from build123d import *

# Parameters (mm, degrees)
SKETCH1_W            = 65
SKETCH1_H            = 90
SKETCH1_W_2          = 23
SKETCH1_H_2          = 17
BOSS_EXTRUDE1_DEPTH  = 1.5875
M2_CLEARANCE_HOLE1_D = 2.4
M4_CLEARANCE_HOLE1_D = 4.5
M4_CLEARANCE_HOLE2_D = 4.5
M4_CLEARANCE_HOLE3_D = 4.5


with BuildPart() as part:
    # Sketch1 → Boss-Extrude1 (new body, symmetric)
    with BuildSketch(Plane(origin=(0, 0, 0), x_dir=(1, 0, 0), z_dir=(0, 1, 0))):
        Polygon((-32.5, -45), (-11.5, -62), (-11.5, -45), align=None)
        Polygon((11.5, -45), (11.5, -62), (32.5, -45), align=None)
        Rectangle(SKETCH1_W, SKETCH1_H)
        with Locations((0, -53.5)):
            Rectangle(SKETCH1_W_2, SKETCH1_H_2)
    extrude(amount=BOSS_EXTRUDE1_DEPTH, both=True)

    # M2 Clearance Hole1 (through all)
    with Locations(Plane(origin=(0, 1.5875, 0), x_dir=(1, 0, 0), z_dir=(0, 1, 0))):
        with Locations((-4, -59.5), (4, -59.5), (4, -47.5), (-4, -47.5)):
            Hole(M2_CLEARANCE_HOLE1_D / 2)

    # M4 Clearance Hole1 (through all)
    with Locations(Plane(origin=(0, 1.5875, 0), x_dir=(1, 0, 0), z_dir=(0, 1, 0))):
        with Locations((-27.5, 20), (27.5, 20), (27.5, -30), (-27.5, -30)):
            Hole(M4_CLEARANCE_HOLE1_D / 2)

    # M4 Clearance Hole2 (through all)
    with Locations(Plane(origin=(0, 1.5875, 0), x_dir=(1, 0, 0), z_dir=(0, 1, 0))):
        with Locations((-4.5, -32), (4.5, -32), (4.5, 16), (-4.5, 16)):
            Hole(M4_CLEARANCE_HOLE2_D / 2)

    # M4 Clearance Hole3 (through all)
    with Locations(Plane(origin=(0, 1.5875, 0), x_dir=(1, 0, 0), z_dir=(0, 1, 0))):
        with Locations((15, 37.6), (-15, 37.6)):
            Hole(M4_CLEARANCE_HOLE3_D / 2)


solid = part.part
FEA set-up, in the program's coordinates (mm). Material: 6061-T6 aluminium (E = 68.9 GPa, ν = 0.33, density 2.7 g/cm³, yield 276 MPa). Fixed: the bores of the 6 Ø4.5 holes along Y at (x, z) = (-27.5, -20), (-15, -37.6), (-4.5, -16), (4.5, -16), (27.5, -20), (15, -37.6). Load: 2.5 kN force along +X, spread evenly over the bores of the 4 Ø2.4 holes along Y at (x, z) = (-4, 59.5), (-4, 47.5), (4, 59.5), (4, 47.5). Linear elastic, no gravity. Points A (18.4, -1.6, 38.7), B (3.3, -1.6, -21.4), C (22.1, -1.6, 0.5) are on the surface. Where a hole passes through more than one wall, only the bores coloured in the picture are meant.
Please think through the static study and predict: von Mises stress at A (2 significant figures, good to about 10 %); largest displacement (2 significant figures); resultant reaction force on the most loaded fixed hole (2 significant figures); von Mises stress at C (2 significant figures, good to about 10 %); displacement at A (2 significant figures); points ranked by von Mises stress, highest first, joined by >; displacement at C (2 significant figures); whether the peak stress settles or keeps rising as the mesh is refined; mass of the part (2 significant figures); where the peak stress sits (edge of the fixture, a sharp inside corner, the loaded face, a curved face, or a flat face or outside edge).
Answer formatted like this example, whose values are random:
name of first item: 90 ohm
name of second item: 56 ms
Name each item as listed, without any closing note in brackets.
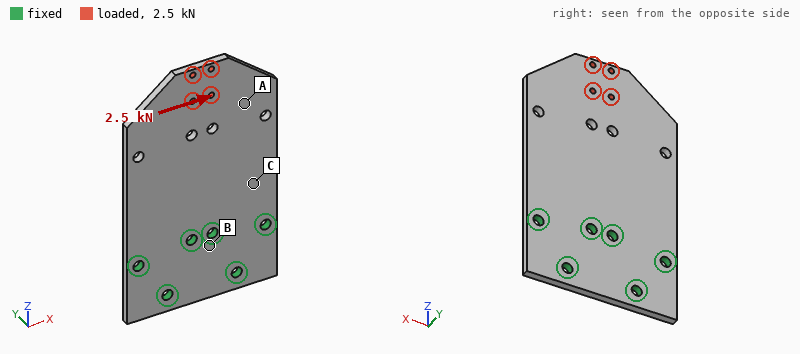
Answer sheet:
von Mises stress at A: 24 MPa
largest displacement: 0.12 mm
resultant reaction force on the most loaded fixed hole: 2.9 kN
von Mises stress at C: 44 MPa
displacement at A: 0.083 mm
points ranked by von Mises stress, highest first, joined by >: C > A > B
displacement at C: 0.022 mm
whether the peak stress settles or keeps rising as the mesh is refined: keeps rising
mass of the part: 55 g
where the peak stress sits: edge of the fixture
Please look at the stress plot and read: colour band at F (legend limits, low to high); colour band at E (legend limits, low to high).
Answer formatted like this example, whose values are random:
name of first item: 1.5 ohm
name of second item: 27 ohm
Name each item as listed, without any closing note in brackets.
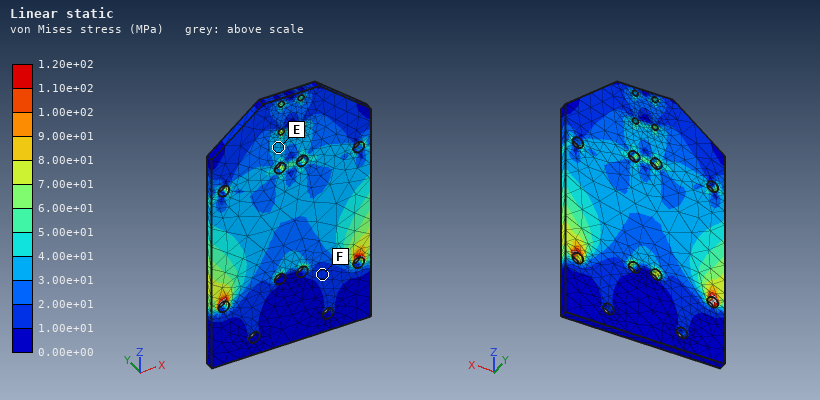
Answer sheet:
colour band at F: 1.00e+01 to 2.00e+01 MPa
colour band at E: 3.00e+01 to 4.00e+01 MPa
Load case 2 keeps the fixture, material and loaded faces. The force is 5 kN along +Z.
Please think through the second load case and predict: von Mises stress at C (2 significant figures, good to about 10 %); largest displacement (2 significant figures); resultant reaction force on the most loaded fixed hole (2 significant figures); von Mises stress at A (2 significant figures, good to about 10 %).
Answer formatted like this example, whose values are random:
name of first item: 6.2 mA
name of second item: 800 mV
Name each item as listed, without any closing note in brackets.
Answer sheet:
von Mises stress at C: 23 MPa
largest displacement: 44 µm
resultant reaction force on the most loaded fixed hole: 1.2 kN
von Mises stress at A: 24 MPa
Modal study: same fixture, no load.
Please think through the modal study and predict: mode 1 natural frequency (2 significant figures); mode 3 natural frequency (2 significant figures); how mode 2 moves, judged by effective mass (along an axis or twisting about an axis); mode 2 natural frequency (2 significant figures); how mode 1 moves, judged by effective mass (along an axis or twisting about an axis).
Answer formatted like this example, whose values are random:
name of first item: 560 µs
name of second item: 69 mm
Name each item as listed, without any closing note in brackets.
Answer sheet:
mode 1 natural frequency: 500 Hz
mode 3 natural frequency: 2700 Hz
how mode 2 moves, judged by effective mass: twisting about Z
mode 2 natural frequency: 1400 Hz
how mode 1 moves, judged by effective mass: along Y
